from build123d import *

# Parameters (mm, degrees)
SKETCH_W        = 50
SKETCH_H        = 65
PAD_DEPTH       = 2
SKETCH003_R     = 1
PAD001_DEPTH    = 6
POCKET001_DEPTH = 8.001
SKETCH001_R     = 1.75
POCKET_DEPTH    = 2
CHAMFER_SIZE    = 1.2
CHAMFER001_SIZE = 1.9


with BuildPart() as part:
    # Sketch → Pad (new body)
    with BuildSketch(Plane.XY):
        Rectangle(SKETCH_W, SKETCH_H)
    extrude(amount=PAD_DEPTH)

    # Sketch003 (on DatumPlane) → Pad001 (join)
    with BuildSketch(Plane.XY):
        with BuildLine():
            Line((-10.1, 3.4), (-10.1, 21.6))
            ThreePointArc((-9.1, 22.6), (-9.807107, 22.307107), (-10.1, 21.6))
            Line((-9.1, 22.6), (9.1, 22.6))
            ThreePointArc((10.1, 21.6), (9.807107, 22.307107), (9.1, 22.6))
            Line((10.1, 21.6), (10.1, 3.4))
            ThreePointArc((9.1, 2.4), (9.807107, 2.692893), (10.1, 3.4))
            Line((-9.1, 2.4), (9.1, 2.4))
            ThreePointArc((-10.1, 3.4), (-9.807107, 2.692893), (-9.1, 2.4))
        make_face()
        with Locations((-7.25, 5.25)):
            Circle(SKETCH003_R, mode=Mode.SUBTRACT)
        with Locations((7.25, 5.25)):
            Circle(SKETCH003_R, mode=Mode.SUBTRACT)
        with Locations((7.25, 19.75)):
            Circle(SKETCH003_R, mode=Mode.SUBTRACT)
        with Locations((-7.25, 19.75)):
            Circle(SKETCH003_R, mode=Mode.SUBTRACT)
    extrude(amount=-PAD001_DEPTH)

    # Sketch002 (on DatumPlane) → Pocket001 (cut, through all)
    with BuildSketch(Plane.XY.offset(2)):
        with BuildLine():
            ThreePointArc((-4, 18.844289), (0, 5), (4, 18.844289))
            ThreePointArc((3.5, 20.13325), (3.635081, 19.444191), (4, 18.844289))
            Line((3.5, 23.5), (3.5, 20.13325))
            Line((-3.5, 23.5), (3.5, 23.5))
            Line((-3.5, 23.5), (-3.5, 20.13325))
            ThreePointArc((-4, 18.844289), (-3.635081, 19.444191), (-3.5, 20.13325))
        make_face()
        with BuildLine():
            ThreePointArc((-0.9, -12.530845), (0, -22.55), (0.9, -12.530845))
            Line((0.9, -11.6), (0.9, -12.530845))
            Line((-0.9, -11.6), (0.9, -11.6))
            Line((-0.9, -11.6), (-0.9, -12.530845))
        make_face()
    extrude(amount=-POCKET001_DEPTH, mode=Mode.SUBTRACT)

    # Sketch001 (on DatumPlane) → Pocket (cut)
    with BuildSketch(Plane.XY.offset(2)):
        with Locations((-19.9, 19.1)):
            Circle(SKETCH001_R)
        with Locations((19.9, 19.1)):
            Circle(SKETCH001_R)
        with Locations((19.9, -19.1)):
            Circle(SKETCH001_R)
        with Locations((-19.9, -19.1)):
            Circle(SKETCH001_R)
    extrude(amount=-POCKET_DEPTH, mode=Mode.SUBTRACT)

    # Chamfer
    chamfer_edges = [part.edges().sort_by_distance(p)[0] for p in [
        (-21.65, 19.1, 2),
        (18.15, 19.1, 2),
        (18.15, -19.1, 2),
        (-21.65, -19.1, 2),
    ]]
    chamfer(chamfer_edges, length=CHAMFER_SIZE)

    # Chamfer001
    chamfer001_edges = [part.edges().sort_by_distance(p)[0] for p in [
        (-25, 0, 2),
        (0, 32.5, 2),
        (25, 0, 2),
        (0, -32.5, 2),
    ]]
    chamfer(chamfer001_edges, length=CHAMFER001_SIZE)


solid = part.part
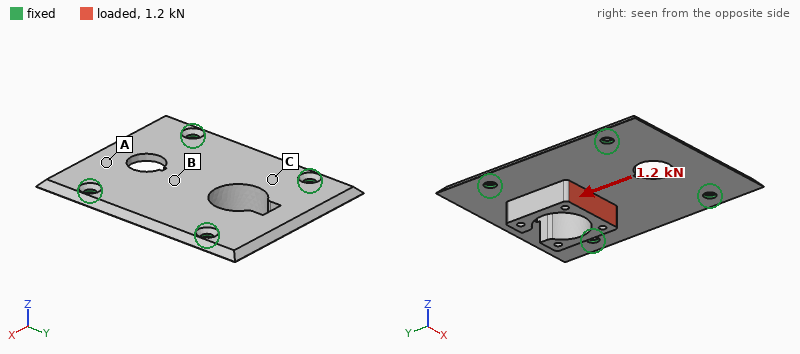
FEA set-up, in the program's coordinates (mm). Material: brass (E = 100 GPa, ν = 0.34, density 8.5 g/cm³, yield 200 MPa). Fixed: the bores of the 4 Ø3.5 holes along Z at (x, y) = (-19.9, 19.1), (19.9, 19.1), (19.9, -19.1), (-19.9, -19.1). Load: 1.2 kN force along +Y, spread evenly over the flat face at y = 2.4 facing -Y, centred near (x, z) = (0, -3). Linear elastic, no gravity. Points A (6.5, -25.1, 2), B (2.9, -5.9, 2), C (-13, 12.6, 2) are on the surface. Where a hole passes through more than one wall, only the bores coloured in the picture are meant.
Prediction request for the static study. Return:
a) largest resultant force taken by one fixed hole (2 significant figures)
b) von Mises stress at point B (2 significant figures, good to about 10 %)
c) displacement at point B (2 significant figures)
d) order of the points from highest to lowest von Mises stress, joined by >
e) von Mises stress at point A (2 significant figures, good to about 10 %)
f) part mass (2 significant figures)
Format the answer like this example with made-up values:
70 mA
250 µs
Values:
440 N
30 MPa
45 µm
B > A > C
15 MPa
56 g
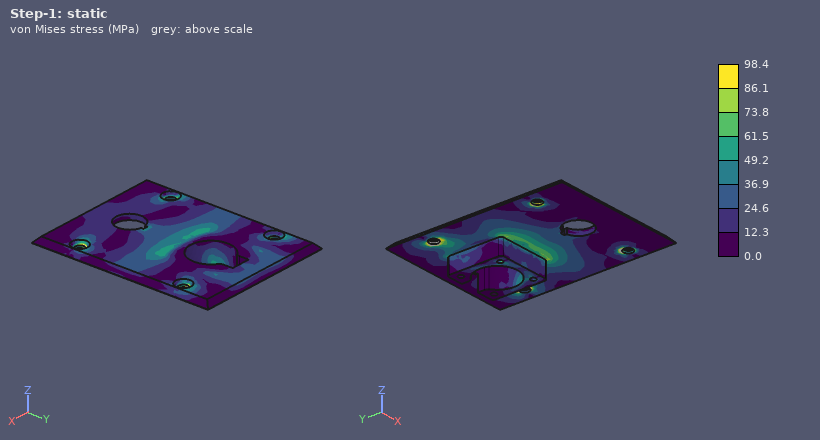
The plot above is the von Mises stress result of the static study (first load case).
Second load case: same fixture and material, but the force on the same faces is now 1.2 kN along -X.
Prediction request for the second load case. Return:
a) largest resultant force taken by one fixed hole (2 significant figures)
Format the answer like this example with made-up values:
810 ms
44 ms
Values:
370 N
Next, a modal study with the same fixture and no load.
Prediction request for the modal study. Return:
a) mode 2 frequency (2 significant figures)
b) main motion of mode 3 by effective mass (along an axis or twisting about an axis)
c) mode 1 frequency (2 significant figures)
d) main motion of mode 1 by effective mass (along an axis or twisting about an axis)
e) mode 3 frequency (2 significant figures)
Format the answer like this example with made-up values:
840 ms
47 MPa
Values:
3300 Hz
along Z
2800 Hz
along Z
3500 Hz
